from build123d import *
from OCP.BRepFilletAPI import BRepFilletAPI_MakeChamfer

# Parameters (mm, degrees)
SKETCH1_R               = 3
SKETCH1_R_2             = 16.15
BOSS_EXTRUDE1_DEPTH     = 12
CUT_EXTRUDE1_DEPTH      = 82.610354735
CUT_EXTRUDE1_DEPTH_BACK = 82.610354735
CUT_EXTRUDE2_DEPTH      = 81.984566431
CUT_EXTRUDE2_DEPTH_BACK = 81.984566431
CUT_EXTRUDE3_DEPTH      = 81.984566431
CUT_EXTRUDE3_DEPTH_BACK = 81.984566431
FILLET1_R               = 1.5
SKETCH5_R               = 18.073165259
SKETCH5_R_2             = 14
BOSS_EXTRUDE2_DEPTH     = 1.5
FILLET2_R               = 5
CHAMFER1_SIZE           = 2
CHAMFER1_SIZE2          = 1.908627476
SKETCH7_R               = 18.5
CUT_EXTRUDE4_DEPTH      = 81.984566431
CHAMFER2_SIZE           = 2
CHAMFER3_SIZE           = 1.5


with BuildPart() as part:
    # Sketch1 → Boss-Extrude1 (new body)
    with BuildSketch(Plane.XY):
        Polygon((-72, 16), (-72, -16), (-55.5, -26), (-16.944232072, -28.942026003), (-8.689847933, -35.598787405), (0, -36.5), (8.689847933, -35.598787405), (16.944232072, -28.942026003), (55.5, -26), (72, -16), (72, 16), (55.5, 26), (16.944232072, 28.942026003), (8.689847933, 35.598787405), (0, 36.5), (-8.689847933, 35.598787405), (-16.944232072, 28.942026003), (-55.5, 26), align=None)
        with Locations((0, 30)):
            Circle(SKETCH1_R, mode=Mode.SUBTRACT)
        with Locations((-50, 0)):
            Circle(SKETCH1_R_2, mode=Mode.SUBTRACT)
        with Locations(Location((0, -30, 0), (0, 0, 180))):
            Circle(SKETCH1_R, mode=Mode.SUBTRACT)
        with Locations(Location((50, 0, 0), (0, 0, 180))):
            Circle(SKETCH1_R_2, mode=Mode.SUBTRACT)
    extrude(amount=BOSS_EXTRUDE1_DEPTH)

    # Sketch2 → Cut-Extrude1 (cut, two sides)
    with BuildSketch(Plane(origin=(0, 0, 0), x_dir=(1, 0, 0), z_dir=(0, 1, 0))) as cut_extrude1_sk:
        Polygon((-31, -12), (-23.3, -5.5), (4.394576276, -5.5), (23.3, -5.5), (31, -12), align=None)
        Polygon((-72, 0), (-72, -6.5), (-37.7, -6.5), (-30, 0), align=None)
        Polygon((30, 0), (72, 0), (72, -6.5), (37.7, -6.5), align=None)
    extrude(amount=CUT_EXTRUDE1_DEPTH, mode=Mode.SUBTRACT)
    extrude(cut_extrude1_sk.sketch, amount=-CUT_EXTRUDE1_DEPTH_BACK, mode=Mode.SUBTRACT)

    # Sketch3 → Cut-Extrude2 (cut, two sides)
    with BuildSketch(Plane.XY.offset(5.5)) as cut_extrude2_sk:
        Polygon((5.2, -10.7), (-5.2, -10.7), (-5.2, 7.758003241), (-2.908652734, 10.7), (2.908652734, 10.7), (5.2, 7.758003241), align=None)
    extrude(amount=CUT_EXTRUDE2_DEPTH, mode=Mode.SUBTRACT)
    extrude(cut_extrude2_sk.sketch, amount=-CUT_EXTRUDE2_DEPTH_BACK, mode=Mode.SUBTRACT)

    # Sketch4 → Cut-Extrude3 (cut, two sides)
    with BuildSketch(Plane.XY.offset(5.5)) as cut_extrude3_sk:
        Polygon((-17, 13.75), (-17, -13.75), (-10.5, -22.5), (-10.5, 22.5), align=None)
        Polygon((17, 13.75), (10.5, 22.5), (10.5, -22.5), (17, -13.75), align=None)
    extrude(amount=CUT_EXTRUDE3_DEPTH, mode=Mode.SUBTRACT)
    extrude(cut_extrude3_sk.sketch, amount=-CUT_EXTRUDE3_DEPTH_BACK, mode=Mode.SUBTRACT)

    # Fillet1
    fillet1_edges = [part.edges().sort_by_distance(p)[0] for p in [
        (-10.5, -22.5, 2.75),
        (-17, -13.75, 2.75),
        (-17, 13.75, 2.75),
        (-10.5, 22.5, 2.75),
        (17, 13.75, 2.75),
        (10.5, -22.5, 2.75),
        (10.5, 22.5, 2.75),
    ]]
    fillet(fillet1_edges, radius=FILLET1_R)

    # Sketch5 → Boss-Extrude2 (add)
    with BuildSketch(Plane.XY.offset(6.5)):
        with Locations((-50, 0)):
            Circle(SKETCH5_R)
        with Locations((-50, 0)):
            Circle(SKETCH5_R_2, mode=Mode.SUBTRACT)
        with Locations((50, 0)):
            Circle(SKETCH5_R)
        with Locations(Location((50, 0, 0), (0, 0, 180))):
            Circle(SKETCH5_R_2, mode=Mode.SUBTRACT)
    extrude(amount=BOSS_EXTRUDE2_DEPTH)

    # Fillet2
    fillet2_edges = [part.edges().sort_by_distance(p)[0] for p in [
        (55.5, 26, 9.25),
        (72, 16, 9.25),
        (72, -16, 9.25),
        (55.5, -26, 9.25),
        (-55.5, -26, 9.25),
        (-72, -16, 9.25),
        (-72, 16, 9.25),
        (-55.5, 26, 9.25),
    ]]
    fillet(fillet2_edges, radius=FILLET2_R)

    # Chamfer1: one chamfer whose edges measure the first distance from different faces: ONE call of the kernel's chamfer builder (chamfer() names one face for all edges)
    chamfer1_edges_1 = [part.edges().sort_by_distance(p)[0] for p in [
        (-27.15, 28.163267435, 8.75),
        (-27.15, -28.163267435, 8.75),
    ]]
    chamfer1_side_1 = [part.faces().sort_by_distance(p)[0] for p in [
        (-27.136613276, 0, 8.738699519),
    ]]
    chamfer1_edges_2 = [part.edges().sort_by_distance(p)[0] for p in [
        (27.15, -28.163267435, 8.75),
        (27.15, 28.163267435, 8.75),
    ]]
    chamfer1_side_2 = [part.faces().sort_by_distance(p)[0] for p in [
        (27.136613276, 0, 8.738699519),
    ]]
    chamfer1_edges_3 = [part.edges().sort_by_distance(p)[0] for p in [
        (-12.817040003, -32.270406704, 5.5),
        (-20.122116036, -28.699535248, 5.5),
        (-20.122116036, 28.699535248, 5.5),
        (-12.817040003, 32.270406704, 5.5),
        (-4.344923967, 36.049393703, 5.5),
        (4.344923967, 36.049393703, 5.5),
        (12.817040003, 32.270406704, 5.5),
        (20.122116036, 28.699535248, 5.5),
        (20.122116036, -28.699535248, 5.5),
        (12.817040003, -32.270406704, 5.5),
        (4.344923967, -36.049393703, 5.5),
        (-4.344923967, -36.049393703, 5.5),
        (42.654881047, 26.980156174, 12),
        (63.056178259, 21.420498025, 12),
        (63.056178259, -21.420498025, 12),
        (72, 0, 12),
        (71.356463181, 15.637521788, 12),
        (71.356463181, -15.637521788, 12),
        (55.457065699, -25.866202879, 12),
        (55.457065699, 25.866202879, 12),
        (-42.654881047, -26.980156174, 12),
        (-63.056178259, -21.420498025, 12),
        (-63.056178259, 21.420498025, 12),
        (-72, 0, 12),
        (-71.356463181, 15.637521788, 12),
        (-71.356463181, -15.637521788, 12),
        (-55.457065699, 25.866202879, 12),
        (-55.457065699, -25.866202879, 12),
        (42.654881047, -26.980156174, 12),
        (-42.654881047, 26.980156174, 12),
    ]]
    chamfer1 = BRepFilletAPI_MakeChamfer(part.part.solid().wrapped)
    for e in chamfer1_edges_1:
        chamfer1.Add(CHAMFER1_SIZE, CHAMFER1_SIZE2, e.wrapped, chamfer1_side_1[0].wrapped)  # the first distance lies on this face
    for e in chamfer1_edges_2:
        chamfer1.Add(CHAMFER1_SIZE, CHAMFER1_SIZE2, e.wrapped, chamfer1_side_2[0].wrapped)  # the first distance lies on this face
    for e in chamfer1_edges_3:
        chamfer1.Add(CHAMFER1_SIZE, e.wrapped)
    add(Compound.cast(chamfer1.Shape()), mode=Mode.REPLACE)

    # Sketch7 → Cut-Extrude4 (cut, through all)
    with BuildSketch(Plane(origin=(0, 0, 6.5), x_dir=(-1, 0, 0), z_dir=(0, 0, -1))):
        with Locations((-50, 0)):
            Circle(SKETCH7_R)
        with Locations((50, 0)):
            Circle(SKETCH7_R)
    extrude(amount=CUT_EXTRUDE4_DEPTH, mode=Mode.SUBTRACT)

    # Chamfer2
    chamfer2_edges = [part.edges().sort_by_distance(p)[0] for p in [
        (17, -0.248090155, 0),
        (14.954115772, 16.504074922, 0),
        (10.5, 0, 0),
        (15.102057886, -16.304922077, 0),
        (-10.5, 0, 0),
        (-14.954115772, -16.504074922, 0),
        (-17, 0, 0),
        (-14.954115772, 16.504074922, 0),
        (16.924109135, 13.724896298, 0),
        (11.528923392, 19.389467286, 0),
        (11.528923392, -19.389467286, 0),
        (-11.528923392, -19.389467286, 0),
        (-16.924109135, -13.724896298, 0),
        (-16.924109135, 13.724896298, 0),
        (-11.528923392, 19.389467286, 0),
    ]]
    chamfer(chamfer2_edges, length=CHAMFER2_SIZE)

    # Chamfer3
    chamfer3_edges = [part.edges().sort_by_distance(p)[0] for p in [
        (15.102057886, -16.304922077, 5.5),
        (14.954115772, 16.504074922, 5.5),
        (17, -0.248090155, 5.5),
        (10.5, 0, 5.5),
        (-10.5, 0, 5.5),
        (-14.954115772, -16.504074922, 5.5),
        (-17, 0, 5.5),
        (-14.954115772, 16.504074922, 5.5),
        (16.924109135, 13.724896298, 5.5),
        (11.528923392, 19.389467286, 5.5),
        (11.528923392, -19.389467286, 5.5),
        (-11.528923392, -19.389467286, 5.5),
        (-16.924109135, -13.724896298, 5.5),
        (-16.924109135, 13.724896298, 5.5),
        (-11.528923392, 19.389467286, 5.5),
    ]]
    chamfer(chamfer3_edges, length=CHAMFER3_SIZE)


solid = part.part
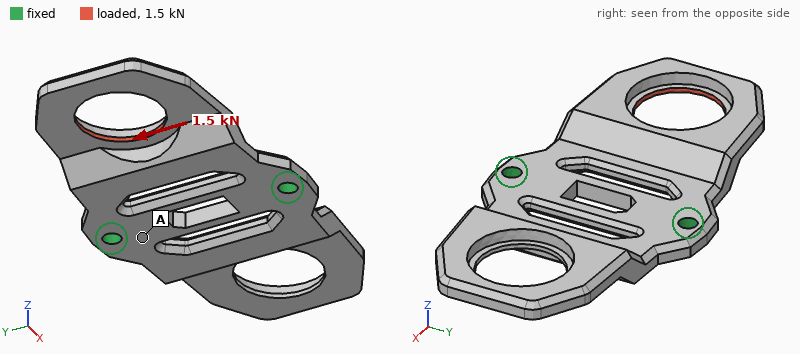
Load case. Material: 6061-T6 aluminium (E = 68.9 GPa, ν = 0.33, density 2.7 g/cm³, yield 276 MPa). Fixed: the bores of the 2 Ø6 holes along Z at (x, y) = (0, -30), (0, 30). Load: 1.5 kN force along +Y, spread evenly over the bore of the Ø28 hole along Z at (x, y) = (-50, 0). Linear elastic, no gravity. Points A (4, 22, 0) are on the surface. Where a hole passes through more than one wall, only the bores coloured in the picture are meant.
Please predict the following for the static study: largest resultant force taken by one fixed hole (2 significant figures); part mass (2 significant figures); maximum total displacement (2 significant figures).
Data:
1.4 kN
93 g
73 µm
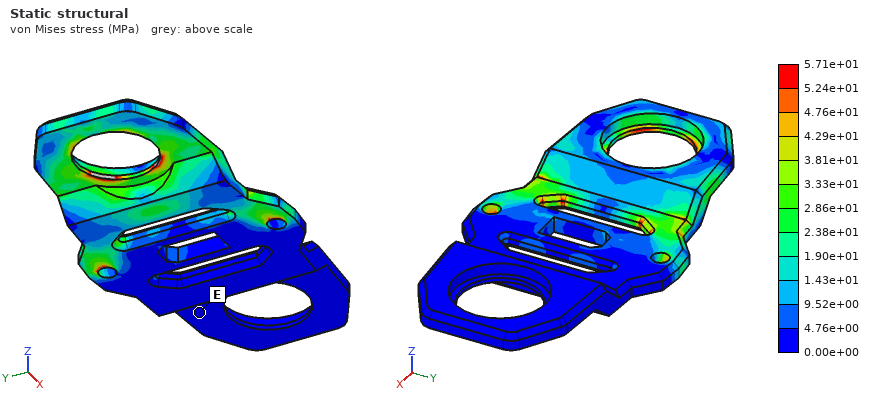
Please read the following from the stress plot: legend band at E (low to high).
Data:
0.00e+00 to 4.76e+00 MPa
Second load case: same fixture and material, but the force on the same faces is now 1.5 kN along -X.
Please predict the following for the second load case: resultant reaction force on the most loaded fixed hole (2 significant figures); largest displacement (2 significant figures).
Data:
780 N
0.36 mm
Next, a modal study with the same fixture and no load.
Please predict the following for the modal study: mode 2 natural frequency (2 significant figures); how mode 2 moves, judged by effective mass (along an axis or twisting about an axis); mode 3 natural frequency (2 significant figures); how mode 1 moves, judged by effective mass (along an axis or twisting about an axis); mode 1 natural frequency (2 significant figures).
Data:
880 Hz
along Z
3200 Hz
twisting about Y
850 Hz
